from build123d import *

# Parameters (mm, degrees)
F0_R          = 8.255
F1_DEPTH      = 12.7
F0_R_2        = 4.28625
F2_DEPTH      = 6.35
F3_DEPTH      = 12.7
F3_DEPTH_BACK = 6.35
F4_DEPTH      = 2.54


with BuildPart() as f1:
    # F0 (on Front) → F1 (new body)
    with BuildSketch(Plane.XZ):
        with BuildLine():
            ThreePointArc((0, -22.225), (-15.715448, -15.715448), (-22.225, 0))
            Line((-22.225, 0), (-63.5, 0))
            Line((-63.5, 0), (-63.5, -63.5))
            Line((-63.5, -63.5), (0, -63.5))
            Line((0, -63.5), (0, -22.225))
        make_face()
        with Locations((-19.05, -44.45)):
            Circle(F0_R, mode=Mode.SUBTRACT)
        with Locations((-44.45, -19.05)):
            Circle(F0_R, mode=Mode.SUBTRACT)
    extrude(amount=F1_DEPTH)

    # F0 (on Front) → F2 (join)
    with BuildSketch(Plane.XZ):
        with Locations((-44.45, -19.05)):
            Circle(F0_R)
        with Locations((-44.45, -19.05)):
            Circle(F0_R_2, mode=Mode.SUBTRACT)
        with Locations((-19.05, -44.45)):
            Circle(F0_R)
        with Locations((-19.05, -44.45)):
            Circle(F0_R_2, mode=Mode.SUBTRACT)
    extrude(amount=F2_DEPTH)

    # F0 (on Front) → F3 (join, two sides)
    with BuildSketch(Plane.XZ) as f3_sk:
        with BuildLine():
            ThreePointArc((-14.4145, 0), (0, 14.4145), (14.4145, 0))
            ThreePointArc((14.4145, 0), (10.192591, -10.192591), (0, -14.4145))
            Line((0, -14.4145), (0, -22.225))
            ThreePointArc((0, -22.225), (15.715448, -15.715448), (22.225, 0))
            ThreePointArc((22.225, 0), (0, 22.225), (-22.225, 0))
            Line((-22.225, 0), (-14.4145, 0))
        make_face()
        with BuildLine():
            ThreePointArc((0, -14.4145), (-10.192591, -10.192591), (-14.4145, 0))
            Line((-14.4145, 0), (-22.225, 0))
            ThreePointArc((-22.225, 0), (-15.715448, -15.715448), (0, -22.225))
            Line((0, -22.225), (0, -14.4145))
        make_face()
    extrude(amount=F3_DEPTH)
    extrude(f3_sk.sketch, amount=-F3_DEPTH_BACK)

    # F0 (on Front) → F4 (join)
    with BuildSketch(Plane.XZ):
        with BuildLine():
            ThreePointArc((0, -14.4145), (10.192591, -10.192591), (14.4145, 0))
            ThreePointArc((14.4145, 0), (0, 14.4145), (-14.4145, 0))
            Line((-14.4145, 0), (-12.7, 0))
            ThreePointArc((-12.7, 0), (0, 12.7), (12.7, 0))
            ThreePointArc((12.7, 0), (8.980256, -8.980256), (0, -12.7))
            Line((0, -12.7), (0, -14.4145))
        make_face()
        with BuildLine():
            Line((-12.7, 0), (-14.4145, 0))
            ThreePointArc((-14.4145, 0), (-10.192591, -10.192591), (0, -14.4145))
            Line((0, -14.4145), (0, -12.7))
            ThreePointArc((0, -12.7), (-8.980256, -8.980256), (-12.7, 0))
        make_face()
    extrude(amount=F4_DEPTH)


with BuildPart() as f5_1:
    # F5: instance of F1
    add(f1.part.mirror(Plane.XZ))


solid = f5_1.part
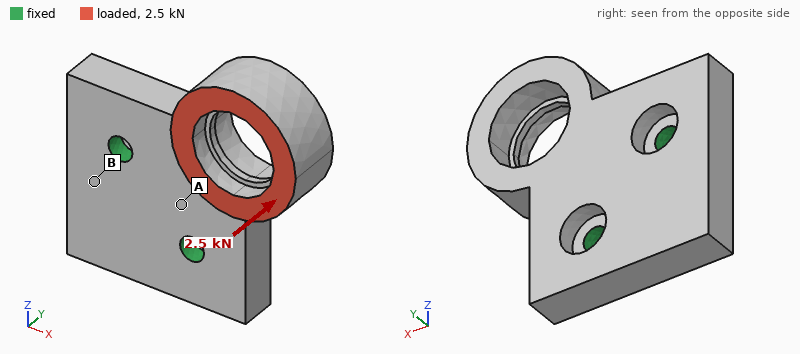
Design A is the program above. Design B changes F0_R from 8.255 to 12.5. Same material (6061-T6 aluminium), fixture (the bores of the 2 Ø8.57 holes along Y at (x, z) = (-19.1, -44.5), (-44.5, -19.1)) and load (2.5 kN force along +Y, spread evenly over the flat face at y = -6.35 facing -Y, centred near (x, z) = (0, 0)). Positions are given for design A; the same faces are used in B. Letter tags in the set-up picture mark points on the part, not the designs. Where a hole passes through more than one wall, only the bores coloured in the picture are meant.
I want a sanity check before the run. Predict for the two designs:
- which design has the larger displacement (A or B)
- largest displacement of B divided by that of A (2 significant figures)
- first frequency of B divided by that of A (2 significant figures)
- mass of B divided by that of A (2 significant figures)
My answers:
B
1.2
0.92
0.94
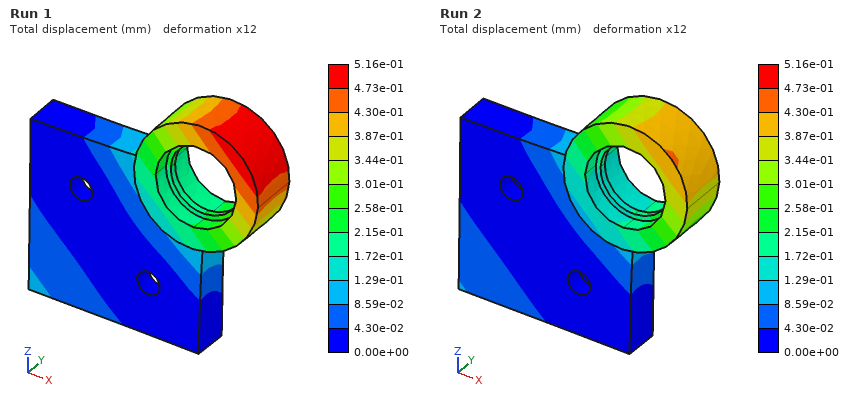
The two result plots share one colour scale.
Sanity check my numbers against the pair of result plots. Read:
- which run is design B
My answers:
Run 1
